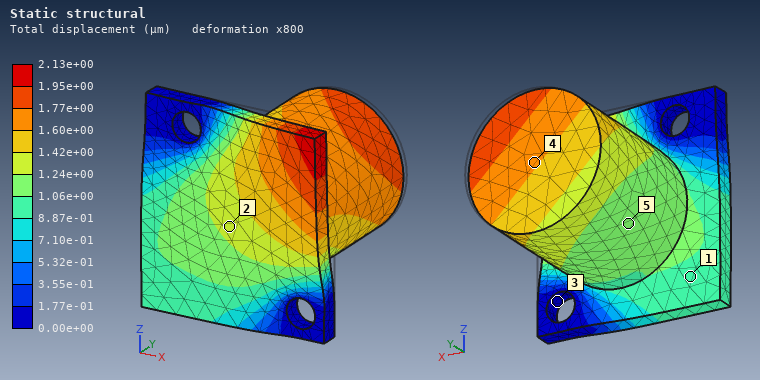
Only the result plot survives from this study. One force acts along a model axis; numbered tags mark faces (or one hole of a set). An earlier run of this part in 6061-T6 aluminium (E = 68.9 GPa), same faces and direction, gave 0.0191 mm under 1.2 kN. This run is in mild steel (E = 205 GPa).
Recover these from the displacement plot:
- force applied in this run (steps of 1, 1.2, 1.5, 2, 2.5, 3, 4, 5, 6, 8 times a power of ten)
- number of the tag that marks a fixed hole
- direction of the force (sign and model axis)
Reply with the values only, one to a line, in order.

400 N
3
-Y
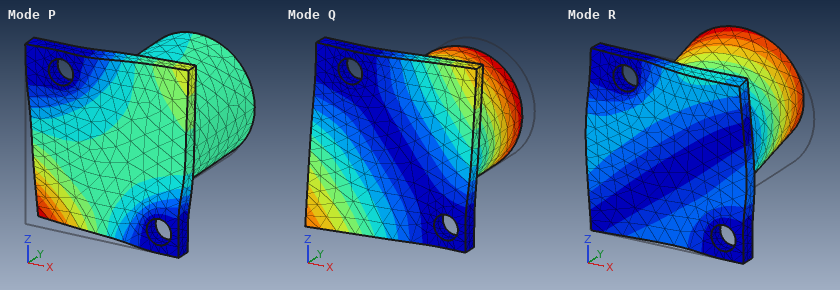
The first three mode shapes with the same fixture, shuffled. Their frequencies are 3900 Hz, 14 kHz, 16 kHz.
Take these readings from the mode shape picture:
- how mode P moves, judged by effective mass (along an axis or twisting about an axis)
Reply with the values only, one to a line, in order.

along Y
